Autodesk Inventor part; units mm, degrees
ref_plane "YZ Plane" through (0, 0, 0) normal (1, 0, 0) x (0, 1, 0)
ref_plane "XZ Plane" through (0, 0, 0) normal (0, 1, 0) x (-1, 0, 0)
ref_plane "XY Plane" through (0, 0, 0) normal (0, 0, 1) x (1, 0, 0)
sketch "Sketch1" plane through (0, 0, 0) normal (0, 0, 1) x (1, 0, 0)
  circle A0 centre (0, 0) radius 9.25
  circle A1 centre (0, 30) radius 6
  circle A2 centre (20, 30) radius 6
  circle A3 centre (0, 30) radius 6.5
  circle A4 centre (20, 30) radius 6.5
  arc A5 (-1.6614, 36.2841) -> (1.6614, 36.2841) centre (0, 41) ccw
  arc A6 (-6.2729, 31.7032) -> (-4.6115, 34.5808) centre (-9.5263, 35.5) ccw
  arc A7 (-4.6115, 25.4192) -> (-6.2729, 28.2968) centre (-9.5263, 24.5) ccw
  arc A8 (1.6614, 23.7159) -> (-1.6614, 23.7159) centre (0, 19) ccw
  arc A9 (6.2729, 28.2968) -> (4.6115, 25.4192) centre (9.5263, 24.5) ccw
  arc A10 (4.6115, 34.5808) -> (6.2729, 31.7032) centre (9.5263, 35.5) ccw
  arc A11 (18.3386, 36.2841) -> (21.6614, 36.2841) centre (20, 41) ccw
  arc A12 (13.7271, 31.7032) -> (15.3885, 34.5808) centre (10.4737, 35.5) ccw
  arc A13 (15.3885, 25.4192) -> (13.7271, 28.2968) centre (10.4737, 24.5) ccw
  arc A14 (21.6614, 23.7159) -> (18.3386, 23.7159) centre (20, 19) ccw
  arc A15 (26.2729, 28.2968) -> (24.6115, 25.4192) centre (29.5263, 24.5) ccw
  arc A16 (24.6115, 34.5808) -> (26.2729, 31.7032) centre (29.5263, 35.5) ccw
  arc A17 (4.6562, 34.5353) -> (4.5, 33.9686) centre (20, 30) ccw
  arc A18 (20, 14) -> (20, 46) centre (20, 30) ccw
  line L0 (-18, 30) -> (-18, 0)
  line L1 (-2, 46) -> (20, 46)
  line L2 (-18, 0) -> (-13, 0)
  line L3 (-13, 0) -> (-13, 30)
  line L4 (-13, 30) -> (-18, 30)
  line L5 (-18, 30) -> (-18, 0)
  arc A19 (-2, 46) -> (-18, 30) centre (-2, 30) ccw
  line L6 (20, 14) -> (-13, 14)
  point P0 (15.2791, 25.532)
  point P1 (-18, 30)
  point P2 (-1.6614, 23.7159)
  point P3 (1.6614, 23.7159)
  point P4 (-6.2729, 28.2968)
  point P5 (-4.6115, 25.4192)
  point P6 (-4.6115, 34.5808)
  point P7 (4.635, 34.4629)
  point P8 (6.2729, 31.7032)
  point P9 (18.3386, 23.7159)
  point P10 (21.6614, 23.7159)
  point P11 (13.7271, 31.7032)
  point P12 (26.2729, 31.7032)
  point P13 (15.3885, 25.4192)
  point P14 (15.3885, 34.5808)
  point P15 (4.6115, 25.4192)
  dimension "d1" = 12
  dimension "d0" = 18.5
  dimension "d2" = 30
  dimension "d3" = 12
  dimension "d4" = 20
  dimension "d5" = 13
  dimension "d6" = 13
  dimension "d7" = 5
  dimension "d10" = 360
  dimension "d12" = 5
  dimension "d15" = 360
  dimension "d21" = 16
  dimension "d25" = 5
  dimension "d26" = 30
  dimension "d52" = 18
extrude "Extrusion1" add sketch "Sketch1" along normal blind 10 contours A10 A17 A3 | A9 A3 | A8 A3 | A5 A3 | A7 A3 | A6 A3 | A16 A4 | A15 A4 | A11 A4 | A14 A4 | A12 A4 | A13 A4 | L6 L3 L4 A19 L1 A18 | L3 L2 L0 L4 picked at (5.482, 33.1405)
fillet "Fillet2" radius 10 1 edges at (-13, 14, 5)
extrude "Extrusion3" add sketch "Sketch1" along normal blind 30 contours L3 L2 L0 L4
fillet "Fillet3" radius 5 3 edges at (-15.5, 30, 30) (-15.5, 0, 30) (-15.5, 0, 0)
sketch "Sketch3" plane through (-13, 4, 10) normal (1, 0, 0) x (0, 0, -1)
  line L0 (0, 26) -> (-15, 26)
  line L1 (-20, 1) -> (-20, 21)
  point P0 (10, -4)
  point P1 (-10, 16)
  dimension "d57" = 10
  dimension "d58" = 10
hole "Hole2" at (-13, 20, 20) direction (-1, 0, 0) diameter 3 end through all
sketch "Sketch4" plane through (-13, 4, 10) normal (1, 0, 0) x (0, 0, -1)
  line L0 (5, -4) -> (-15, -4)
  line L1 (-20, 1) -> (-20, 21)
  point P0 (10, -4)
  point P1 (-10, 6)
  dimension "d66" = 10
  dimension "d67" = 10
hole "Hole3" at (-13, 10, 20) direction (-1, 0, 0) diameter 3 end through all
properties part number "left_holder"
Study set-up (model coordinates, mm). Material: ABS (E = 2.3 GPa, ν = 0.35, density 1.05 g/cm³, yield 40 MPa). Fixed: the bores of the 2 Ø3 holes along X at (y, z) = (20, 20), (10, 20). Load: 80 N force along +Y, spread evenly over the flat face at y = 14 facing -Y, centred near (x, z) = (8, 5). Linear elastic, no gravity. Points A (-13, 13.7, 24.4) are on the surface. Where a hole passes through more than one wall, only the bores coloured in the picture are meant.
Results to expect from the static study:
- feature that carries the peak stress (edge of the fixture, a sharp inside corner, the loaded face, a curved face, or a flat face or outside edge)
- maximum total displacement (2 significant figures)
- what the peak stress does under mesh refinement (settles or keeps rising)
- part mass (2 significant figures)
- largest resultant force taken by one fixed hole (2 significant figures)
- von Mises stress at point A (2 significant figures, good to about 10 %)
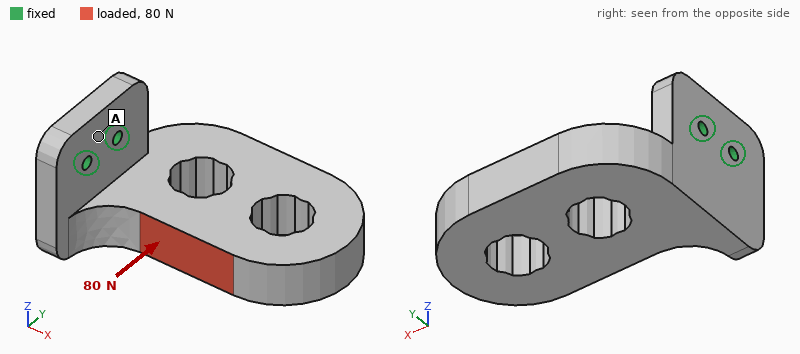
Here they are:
edge of the fixture
0.86 mm
keeps rising
18 g
160 N
2.2 MPa
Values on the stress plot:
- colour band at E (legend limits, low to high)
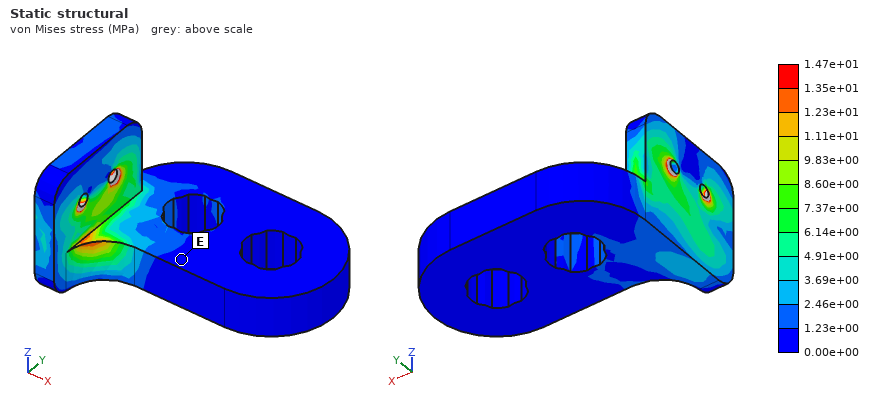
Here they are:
0.00e+00 to 1.23e+00 MPa
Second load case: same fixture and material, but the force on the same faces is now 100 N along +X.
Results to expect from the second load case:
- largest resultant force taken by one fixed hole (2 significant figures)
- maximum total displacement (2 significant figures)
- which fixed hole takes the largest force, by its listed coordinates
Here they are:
56 N
0.88 mm
(10, 20)
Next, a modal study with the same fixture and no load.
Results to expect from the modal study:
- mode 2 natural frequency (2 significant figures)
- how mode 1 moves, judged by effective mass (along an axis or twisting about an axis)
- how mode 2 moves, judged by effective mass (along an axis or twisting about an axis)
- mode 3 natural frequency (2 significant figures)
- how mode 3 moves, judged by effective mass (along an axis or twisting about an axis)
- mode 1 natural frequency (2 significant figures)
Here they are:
480 Hz
along Z
along Y
1600 Hz
along X
310 Hz
